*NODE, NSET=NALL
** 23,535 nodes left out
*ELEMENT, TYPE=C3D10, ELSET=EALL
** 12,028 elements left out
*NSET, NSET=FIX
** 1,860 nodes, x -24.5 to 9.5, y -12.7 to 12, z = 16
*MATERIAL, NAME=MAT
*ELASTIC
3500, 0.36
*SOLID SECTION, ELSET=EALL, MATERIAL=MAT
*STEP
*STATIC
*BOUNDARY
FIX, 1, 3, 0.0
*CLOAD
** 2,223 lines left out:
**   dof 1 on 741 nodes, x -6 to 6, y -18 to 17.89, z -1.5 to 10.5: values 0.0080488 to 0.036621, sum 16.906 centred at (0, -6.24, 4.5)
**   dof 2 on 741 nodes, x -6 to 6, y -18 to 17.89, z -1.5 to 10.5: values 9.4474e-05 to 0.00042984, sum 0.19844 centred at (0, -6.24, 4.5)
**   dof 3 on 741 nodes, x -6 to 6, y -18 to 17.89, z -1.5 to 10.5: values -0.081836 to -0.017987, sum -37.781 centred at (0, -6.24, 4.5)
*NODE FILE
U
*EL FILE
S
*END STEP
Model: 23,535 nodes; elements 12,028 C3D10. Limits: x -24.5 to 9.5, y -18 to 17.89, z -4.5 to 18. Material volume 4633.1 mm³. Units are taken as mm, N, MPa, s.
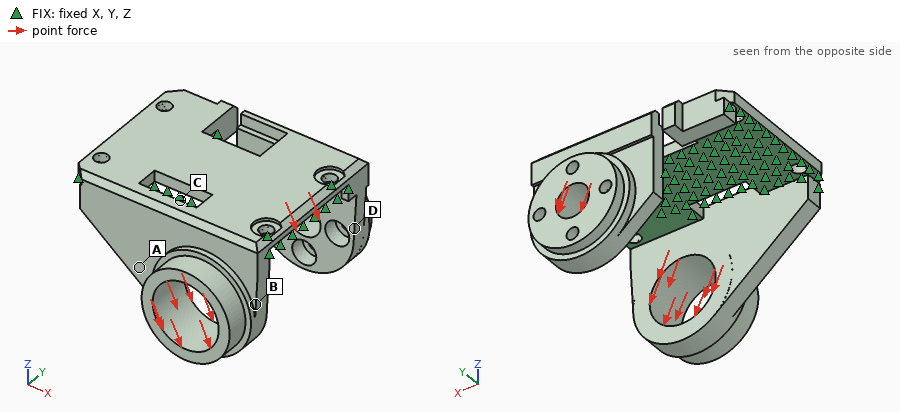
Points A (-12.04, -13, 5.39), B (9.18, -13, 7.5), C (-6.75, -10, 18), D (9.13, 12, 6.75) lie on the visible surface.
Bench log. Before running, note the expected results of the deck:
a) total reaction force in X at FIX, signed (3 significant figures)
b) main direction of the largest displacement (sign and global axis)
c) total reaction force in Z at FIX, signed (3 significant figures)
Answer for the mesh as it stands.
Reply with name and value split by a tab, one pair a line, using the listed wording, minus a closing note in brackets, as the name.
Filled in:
total reaction force in X at FIX, signed	-16.9 N
main direction of the largest displacement	+Y
total reaction force in Z at FIX, signed	37.8 N
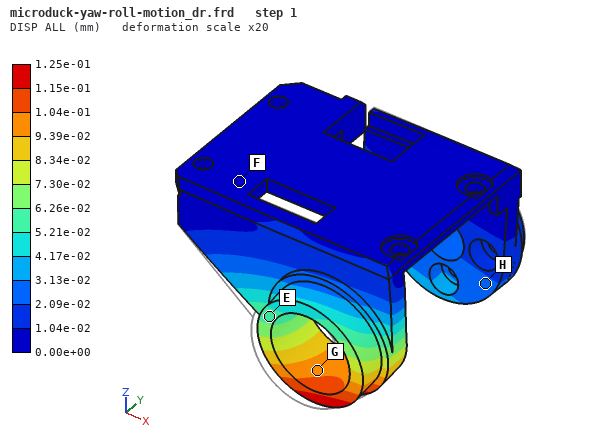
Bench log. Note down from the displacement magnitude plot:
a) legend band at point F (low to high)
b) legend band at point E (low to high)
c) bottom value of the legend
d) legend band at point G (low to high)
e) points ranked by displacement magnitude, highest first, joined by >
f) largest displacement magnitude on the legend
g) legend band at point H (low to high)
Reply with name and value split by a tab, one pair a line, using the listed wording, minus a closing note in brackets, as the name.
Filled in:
legend band at point F	0.00e+00 to 1.04e-02 mm
legend band at point E	5.21e-02 to 6.26e-02 mm
bottom value of the legend	0.00e+00 mm
legend band at point G	9.39e-02 to 1.04e-01 mm
points ranked by displacement magnitude, highest first, joined by >	G > E > H > F
largest displacement magnitude on the legend	1.25e-01 mm
legend band at point H	2.09e-02 to 3.13e-02 mm
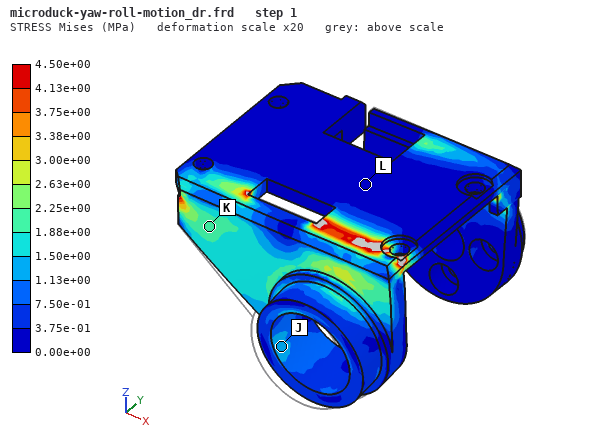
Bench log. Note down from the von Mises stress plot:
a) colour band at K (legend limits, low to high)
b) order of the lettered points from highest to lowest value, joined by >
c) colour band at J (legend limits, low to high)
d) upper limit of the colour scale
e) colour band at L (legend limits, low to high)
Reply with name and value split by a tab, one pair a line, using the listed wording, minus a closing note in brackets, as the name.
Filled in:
colour band at K	1.88e+00 to 2.25e+00 MPa
order of the lettered points from highest to lowest value, joined by >	K > J > L
colour band at J	1.13e+00 to 1.50e+00 MPa
upper limit of the colour scale	4.50e+00 MPa
colour band at L	0.00e+00 to 3.75e-01 MPa
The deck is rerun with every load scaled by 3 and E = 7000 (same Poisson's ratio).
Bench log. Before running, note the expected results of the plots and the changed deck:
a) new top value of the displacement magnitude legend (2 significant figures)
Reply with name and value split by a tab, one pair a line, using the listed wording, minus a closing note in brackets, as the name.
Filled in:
new top value of the displacement magnitude legend	0.19 mm
